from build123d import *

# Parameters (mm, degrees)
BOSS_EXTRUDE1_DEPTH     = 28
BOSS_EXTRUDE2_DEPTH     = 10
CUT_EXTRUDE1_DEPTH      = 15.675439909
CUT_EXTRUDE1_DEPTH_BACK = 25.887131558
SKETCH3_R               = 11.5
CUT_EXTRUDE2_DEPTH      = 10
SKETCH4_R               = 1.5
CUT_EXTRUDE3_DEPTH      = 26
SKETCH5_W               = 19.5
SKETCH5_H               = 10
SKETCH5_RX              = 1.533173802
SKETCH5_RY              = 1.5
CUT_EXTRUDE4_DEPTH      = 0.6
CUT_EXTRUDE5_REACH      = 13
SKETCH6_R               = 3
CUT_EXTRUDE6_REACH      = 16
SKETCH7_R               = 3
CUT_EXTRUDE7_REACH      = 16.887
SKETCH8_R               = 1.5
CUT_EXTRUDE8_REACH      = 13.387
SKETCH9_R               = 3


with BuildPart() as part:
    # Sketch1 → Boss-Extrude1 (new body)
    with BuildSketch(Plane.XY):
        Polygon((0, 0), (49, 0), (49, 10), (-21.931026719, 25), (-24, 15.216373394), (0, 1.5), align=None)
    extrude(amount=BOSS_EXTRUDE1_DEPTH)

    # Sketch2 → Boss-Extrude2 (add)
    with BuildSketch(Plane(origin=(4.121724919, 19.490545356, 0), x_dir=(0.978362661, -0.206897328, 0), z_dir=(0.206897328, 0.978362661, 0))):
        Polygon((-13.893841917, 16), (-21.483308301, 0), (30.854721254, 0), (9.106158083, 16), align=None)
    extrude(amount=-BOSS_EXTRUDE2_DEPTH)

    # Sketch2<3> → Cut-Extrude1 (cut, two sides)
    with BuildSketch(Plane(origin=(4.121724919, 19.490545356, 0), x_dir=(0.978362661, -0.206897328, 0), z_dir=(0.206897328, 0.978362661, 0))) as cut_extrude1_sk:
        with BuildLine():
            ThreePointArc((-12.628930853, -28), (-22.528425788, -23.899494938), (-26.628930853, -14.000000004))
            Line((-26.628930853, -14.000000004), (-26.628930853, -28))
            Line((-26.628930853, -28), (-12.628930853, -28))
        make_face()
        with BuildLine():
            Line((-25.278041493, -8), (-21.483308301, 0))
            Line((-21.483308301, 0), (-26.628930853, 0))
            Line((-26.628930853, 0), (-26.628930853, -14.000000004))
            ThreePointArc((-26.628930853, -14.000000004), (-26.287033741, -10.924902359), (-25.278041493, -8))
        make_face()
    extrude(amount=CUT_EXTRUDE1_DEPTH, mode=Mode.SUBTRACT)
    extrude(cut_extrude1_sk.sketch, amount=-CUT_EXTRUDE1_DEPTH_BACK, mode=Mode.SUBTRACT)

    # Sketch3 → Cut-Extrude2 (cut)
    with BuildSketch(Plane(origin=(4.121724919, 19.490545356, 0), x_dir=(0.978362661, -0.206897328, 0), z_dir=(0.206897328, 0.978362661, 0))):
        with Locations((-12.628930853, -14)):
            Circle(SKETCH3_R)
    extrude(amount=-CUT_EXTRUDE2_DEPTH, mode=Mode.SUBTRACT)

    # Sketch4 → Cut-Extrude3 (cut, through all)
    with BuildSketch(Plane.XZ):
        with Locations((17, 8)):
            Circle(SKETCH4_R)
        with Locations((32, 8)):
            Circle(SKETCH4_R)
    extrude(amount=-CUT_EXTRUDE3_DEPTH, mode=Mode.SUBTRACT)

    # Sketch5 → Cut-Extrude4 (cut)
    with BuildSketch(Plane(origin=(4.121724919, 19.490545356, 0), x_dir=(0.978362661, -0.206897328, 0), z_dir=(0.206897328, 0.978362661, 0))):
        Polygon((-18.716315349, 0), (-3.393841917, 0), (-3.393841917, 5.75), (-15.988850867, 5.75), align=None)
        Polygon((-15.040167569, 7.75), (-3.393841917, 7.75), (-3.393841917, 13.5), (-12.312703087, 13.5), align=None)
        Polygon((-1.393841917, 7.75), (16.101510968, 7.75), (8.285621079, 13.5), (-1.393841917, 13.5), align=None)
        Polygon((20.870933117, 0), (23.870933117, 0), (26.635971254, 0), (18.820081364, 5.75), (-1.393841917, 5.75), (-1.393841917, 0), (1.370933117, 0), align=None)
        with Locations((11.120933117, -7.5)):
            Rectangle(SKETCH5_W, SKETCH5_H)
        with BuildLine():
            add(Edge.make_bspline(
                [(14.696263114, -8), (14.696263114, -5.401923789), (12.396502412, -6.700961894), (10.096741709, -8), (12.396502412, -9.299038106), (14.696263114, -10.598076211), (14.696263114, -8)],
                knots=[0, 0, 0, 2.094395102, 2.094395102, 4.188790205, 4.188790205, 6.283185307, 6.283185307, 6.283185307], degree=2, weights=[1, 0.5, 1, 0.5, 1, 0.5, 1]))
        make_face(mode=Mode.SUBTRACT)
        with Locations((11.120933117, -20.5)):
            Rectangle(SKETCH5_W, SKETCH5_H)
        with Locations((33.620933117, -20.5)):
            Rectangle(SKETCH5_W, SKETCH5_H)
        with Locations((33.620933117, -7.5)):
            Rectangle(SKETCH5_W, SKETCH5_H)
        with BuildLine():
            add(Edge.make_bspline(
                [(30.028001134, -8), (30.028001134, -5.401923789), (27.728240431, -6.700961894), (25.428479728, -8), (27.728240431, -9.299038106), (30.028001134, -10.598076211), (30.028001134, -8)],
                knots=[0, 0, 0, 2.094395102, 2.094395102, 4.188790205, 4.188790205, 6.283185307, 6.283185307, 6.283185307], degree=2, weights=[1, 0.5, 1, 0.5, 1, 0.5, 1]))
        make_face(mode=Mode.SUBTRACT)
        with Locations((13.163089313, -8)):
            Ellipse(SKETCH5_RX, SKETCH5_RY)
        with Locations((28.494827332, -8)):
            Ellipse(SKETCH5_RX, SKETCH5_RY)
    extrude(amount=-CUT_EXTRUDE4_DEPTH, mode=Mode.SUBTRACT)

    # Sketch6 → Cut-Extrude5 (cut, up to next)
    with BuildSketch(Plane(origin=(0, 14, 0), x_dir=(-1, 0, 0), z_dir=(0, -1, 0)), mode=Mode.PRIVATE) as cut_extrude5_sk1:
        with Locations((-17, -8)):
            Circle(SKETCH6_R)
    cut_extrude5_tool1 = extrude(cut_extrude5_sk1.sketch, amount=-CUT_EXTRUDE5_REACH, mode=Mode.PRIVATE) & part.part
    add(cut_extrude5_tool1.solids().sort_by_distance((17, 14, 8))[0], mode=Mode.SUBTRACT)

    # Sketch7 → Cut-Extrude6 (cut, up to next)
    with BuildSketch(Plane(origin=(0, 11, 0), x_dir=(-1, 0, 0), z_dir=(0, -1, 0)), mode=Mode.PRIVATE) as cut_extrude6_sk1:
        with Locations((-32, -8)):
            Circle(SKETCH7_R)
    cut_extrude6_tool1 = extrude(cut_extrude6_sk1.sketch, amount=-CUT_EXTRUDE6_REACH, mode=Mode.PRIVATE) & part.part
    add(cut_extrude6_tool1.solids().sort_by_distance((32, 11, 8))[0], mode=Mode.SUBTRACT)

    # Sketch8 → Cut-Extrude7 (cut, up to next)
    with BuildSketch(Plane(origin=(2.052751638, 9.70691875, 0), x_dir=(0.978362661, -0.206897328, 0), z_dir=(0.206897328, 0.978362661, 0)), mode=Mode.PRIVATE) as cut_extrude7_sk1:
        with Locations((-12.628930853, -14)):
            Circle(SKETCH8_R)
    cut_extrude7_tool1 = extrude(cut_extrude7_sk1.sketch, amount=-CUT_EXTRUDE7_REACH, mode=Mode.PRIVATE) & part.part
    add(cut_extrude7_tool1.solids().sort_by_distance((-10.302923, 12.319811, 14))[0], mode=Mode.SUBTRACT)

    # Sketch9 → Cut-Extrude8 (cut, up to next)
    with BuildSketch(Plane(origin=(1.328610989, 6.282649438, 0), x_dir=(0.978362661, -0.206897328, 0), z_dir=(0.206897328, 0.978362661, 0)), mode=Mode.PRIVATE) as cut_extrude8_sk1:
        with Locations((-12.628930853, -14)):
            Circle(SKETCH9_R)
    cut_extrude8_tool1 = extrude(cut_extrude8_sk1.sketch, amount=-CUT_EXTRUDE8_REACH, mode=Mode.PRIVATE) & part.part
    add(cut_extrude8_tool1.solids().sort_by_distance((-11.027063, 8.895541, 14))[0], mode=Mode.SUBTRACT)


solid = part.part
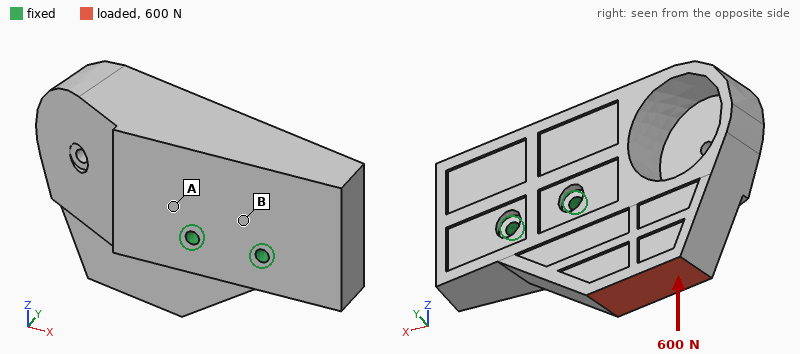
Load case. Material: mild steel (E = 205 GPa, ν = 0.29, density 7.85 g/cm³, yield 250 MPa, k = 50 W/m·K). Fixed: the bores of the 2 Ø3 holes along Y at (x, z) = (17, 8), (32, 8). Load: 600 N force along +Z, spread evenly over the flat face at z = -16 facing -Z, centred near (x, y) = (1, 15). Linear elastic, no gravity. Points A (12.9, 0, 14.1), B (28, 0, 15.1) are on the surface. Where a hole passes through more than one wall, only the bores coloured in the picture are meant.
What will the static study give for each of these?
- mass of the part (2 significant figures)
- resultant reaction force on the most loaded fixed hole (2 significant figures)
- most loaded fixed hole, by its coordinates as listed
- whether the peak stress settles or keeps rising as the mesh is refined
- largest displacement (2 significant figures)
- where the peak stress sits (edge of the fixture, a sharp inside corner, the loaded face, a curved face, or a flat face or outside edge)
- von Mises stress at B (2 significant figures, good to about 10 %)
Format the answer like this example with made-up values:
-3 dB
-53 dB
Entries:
240 g
1.1 kN
(17, 8)
keeps rising
3.0 µm
edge of the fixture
4.1 MPa
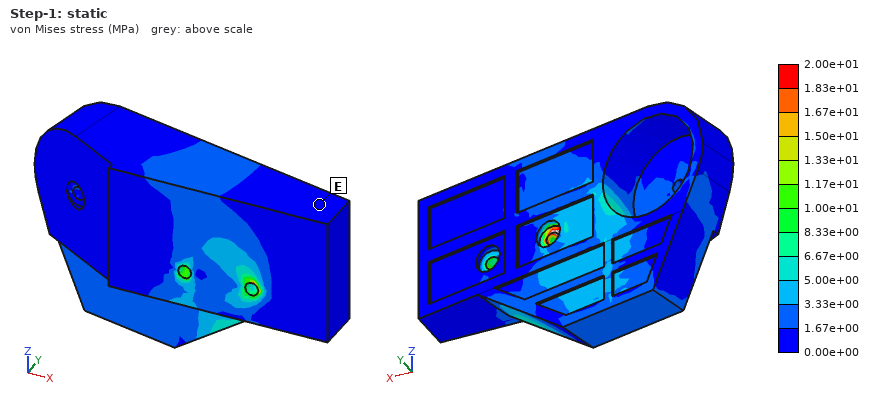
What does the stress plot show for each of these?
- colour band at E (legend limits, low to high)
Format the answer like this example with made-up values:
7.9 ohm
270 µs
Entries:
0.00e+00 to 1.67e+00 MPa
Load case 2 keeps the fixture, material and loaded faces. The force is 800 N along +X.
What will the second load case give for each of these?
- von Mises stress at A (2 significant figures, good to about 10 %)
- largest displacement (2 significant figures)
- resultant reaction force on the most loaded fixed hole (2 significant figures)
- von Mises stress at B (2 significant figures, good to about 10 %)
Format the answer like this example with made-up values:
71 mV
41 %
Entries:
4.3 MPa
4.7 µm
1.3 kN
5.6 MPa
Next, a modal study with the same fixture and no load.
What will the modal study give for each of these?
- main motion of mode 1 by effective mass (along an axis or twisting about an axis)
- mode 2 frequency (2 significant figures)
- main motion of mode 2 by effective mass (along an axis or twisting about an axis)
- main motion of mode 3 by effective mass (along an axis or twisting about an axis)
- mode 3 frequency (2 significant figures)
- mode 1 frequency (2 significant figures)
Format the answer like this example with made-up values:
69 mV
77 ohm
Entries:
along Y
8100 Hz
along Z
twisting about X
9600 Hz
7300 Hz
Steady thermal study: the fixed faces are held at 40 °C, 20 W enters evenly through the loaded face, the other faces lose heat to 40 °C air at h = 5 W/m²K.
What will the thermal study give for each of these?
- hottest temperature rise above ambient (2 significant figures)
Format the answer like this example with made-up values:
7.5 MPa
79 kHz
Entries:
43 K
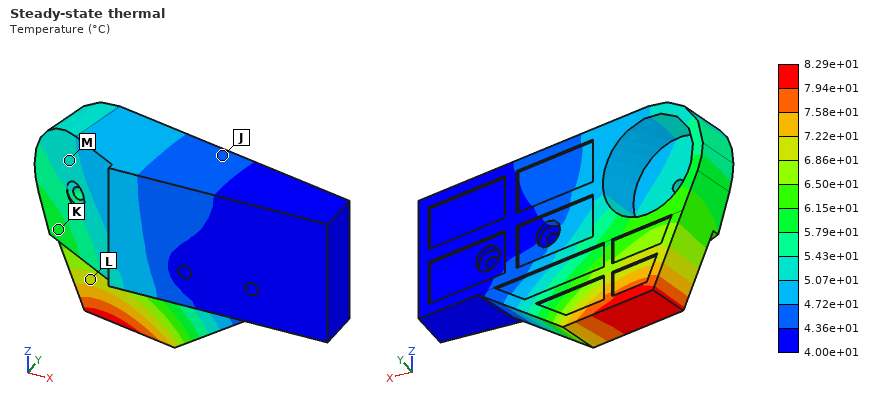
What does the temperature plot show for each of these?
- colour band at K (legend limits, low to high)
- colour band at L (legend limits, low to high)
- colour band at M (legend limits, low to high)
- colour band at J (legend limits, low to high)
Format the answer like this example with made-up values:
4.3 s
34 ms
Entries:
5.79e+01 to 6.15e+01 °C
6.86e+01 to 7.22e+01 °C
5.07e+01 to 5.43e+01 °C
4.36e+01 to 4.72e+01 °C
